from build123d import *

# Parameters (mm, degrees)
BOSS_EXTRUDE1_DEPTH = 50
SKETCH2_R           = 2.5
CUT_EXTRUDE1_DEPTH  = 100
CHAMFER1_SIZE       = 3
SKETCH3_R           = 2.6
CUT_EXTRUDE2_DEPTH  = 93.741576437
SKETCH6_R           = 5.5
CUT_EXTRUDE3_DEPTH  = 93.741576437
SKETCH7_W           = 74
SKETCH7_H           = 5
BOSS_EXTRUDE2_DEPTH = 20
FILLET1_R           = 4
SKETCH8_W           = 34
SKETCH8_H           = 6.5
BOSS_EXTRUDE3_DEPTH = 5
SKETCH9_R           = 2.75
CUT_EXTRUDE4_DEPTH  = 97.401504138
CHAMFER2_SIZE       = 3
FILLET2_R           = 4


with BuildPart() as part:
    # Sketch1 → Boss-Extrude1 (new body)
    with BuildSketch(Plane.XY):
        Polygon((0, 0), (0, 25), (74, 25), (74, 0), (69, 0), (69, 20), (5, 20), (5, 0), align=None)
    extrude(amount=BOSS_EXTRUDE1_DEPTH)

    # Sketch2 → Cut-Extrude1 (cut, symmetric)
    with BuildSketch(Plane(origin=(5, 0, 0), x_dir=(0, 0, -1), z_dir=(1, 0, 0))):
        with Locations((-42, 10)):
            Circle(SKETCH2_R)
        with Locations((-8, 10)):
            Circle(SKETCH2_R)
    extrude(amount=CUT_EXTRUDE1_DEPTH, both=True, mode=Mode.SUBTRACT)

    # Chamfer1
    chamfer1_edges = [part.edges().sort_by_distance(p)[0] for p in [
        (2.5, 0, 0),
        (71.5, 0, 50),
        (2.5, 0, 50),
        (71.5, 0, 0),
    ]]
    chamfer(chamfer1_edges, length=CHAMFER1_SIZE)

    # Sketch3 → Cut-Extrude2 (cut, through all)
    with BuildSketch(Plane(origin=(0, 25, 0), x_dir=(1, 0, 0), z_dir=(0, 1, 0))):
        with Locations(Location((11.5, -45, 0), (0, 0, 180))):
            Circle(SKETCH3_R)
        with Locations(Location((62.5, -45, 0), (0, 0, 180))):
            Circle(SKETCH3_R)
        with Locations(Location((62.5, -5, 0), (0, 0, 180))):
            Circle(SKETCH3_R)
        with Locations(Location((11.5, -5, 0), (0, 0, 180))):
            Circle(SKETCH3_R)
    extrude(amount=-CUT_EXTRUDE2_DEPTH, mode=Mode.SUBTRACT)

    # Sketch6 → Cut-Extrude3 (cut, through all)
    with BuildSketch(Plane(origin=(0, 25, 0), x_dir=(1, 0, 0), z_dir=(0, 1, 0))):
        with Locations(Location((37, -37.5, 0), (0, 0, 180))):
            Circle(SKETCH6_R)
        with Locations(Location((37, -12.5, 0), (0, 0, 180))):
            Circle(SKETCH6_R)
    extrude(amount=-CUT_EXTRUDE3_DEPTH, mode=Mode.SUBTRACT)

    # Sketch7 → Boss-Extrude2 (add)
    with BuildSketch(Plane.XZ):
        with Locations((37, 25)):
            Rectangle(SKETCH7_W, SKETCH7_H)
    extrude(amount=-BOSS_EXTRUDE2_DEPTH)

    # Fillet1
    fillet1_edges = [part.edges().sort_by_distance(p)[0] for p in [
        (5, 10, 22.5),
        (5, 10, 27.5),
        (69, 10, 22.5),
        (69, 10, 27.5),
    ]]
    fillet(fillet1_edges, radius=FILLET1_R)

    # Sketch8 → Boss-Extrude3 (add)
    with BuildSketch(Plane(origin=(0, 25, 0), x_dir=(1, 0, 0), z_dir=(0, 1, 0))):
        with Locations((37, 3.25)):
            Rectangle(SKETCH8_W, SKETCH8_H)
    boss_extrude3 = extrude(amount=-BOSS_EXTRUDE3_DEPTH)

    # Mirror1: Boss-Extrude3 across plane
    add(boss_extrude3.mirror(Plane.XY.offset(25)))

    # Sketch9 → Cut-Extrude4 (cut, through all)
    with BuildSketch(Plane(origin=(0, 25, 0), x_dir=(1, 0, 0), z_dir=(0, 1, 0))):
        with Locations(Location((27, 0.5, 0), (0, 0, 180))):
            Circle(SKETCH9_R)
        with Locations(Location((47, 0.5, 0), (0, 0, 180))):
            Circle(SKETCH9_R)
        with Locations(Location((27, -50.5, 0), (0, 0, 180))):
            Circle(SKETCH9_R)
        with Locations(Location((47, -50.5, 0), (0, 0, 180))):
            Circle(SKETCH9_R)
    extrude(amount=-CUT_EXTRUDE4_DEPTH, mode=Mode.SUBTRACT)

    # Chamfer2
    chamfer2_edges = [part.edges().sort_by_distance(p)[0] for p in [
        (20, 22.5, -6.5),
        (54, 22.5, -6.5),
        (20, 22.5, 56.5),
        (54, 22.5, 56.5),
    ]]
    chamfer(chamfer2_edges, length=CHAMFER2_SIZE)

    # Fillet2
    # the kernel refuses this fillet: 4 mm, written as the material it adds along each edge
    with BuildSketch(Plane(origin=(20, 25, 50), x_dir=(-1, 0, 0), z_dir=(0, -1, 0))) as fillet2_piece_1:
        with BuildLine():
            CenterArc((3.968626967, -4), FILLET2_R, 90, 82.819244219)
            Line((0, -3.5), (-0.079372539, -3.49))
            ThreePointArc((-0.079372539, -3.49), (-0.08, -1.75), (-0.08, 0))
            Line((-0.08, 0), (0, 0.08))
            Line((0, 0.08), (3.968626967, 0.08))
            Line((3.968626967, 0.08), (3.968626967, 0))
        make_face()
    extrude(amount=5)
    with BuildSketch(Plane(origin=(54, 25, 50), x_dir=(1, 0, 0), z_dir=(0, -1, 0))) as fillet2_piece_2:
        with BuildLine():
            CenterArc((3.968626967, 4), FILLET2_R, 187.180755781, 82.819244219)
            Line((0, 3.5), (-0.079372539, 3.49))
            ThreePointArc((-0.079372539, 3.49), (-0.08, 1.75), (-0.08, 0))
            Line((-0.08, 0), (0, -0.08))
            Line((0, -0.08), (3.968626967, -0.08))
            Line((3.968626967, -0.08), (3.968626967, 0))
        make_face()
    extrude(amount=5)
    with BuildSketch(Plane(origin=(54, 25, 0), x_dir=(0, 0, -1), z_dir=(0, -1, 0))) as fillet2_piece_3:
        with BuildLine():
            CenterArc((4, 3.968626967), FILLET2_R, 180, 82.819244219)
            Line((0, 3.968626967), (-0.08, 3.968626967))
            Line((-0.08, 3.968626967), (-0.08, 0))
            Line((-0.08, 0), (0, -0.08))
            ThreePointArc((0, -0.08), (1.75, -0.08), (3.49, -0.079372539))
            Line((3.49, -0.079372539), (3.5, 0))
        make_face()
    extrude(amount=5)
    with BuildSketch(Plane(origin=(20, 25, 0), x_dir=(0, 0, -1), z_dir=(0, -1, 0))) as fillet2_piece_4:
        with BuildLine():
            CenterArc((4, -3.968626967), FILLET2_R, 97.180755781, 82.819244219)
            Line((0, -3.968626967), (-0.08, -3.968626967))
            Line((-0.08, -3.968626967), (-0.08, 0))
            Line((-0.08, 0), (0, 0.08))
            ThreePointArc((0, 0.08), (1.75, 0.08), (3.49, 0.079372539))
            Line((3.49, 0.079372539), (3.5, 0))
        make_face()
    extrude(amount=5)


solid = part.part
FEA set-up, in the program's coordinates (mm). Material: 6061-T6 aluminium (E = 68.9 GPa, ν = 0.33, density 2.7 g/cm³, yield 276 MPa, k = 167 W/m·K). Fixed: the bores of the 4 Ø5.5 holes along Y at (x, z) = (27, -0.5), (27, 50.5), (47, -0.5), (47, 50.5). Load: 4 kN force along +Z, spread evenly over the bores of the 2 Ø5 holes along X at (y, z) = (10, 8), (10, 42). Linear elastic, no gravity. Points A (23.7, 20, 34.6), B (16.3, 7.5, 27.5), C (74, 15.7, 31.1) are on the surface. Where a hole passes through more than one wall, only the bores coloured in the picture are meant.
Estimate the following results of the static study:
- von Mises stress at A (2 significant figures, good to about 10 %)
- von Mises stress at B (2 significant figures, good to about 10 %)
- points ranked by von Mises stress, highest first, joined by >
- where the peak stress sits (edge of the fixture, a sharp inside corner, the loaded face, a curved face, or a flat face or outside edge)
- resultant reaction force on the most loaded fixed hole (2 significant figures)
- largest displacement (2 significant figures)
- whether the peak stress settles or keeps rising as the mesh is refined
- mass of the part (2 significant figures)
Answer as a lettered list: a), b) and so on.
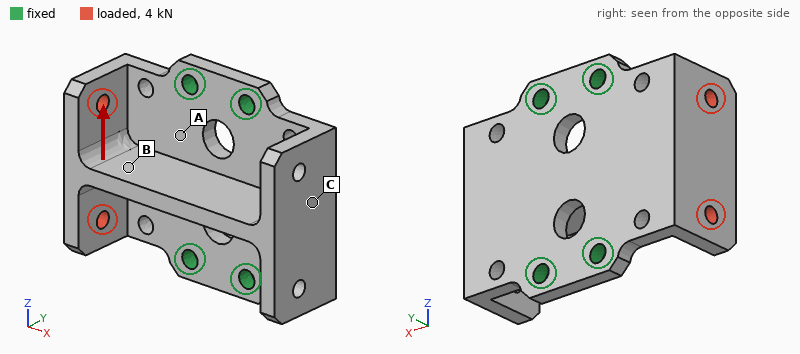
a) 65 MPa
b) 31 MPa
c) A > B > C
d) edge of the fixture
e) 2.8 kN
f) 0.22 mm
g) keeps rising
h) 95 g
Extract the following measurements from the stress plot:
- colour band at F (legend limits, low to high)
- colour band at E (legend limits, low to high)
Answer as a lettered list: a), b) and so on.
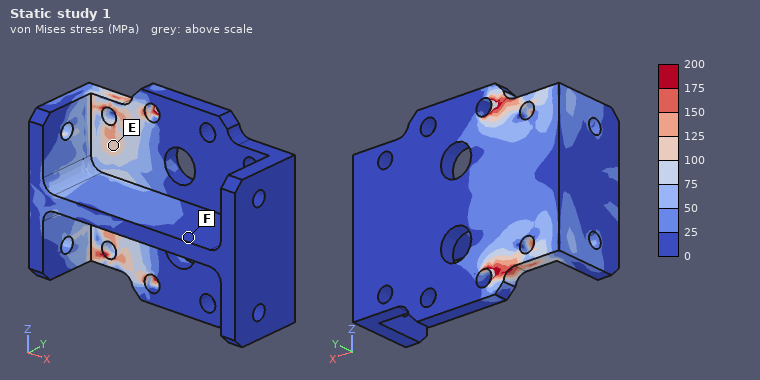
a) 0 to 25 MPa
b) 100 to 125 MPa
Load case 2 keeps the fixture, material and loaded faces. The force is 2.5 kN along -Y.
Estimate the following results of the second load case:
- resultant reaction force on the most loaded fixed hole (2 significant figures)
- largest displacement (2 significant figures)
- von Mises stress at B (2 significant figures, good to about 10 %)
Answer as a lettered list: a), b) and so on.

a) 1.9 kN
b) 0.27 mm
c) 27 MPa
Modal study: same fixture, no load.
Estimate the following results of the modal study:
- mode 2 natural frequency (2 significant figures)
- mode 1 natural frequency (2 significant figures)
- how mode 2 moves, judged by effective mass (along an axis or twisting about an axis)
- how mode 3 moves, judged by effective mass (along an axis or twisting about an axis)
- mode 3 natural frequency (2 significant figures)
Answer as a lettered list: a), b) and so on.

a) 4500 Hz
b) 2700 Hz
c) along Y
d) along Z
e) 4900 Hz
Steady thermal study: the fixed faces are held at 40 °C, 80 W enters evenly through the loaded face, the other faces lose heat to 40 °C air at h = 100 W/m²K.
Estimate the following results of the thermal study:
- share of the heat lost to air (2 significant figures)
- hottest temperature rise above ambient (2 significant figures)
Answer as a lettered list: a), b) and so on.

a) 33 %
b) 63 K
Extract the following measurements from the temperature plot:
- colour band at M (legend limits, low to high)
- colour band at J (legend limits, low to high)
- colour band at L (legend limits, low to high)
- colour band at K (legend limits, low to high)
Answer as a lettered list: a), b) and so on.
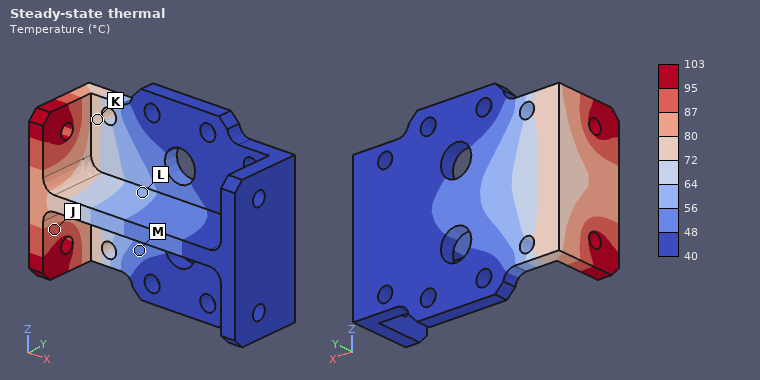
a) 48 to 56 °C
b) 87 to 95 °C
c) 56 to 64 °C
d) 72 to 80 °C
